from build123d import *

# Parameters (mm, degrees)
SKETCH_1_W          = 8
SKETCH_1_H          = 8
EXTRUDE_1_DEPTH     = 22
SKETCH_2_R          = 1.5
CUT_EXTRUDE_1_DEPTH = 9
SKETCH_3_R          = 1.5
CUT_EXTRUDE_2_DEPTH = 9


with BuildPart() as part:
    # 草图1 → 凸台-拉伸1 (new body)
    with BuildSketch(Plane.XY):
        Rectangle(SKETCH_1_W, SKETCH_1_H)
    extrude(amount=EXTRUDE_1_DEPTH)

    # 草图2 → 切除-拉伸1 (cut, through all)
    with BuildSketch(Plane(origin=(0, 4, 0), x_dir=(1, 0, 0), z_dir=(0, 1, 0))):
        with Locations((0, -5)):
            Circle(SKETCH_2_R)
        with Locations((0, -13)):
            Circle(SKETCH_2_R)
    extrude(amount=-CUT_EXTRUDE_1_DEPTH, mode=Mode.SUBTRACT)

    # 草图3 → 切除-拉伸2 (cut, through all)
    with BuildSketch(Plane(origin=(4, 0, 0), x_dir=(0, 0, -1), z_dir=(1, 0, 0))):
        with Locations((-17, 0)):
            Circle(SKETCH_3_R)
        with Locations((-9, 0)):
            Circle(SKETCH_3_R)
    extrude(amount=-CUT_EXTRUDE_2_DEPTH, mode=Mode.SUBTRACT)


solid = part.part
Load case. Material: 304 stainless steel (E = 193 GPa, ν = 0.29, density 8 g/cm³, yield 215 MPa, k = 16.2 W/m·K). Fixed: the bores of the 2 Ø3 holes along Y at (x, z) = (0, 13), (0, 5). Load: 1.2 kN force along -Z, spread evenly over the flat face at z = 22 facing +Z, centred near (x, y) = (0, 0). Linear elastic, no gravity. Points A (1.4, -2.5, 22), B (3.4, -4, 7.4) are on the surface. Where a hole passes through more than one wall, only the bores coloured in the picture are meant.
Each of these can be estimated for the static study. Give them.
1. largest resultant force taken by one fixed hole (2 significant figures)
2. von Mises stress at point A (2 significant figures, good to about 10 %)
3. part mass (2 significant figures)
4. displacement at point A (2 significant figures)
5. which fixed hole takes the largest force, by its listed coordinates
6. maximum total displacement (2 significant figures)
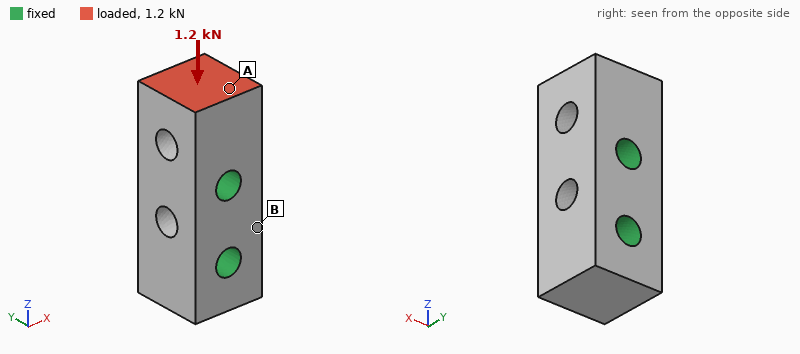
1.1 kN
18 MPa
9.5 g
1.1 µm
(0, 13)
1.3 µm
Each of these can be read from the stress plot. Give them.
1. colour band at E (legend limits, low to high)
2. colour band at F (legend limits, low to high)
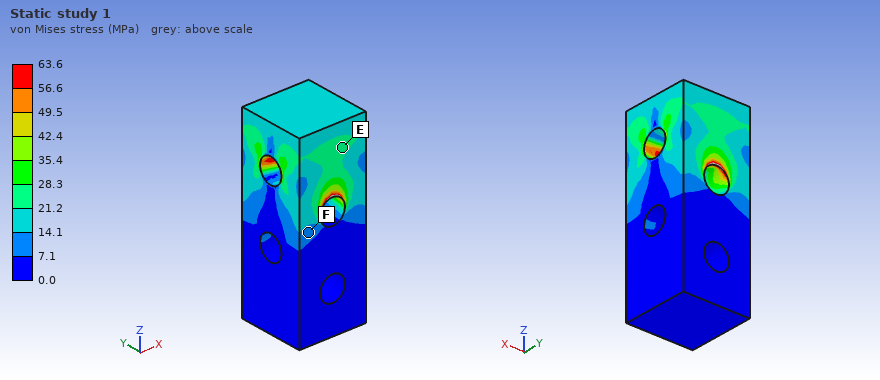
21.2 to 28.3 MPa
7.1 to 14.1 MPa
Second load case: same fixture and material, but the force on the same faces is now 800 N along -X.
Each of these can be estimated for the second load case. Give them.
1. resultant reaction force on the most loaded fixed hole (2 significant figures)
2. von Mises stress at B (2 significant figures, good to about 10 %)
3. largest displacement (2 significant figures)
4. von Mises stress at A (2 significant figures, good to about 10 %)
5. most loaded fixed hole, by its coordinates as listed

1.1 kN
11 MPa
8.4 µm
27 MPa
(0, 13)
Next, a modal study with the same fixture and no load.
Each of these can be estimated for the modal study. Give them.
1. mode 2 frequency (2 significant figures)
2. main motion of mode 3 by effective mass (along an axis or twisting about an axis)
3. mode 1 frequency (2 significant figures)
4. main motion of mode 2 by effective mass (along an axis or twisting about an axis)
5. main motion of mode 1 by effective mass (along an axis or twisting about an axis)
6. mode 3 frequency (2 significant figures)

50 kHz
twisting about Z
44 kHz
along Y
along X
73 kHz
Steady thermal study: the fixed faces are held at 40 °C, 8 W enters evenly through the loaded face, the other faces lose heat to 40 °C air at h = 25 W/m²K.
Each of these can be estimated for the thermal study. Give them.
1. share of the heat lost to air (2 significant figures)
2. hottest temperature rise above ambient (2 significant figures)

4.2 %
79 K
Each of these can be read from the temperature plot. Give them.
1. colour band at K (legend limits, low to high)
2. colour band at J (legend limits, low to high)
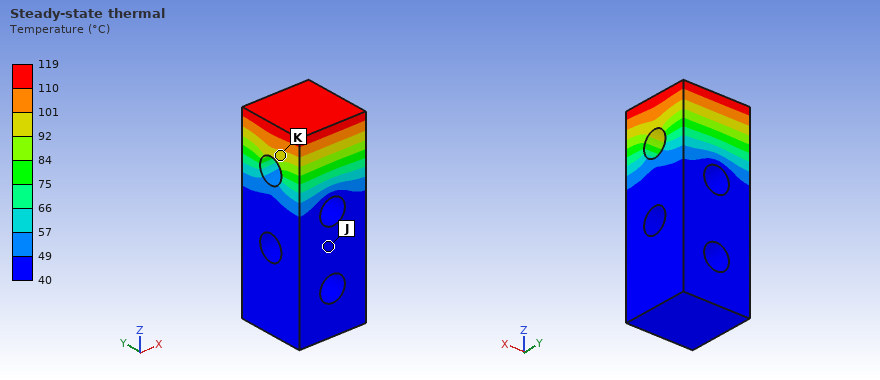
92 to 101 °C
40 to 49 °C
